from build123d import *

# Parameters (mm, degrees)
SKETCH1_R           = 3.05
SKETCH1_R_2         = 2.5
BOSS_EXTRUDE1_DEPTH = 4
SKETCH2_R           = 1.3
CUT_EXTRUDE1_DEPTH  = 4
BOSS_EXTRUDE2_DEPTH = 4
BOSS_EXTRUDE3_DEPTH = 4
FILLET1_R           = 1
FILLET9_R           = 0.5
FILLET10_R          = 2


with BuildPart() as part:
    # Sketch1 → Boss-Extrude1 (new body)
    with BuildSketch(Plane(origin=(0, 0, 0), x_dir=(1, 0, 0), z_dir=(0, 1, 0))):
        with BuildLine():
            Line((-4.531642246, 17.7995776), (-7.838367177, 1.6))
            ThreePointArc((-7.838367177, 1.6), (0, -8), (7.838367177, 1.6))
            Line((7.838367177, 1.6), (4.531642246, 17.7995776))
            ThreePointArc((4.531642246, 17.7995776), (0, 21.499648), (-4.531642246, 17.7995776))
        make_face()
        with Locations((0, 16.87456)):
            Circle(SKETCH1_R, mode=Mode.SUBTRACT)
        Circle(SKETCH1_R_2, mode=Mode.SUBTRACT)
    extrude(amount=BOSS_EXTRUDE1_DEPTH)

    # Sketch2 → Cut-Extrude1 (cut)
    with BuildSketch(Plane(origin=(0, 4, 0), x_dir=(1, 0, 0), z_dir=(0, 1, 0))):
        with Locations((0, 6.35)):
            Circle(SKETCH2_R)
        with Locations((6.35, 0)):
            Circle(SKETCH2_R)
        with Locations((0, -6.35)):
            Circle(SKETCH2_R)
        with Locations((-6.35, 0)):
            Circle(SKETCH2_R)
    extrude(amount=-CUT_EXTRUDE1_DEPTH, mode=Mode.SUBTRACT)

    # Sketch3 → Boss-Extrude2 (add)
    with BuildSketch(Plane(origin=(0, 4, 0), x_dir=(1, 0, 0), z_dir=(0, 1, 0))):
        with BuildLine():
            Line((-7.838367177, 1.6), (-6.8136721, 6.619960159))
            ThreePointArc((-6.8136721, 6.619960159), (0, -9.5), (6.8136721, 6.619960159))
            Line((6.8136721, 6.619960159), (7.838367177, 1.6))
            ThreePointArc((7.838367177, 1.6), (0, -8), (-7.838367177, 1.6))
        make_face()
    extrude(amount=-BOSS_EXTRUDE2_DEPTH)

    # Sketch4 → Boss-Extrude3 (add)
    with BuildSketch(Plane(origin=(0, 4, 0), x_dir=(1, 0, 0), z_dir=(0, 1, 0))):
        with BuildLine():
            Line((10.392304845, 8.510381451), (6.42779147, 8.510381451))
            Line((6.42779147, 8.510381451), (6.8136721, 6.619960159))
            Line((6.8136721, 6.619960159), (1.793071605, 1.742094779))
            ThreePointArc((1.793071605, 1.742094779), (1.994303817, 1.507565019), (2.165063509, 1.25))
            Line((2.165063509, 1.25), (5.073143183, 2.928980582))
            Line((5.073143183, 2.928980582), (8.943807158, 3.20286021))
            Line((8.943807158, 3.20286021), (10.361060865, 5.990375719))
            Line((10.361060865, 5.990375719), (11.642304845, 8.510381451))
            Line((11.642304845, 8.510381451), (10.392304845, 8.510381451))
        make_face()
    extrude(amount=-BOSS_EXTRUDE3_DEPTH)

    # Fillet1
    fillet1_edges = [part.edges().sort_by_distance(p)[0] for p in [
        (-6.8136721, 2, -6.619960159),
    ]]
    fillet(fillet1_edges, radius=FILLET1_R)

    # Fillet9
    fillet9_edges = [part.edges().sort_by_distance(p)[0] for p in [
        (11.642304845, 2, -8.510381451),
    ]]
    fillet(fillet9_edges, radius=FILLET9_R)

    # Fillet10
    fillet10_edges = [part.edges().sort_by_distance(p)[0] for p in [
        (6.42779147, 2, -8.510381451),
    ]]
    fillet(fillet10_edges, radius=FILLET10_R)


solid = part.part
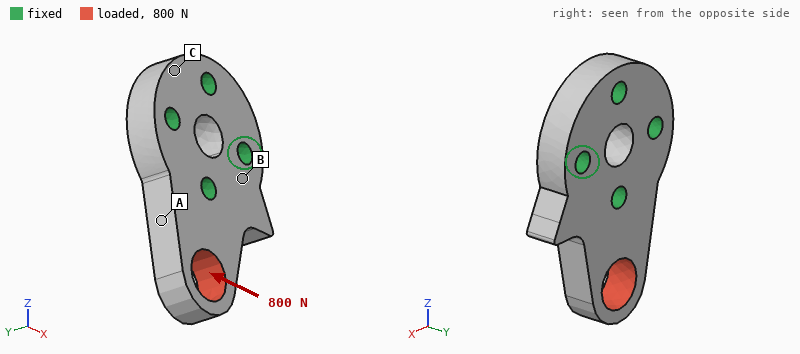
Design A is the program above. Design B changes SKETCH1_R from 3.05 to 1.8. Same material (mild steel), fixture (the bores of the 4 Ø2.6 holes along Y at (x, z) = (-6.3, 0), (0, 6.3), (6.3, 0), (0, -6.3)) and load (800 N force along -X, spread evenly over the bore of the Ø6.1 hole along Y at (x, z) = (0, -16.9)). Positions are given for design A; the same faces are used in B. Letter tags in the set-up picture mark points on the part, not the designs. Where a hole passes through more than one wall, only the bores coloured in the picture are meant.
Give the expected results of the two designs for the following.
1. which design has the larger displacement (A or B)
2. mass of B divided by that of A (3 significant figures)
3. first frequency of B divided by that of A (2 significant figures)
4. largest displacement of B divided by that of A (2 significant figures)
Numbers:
A
1.05
0.89
0.58
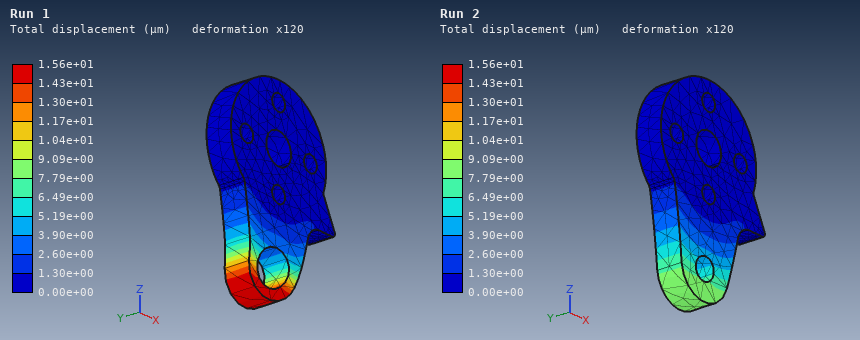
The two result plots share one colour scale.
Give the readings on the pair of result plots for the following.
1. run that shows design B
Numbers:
Run 2
